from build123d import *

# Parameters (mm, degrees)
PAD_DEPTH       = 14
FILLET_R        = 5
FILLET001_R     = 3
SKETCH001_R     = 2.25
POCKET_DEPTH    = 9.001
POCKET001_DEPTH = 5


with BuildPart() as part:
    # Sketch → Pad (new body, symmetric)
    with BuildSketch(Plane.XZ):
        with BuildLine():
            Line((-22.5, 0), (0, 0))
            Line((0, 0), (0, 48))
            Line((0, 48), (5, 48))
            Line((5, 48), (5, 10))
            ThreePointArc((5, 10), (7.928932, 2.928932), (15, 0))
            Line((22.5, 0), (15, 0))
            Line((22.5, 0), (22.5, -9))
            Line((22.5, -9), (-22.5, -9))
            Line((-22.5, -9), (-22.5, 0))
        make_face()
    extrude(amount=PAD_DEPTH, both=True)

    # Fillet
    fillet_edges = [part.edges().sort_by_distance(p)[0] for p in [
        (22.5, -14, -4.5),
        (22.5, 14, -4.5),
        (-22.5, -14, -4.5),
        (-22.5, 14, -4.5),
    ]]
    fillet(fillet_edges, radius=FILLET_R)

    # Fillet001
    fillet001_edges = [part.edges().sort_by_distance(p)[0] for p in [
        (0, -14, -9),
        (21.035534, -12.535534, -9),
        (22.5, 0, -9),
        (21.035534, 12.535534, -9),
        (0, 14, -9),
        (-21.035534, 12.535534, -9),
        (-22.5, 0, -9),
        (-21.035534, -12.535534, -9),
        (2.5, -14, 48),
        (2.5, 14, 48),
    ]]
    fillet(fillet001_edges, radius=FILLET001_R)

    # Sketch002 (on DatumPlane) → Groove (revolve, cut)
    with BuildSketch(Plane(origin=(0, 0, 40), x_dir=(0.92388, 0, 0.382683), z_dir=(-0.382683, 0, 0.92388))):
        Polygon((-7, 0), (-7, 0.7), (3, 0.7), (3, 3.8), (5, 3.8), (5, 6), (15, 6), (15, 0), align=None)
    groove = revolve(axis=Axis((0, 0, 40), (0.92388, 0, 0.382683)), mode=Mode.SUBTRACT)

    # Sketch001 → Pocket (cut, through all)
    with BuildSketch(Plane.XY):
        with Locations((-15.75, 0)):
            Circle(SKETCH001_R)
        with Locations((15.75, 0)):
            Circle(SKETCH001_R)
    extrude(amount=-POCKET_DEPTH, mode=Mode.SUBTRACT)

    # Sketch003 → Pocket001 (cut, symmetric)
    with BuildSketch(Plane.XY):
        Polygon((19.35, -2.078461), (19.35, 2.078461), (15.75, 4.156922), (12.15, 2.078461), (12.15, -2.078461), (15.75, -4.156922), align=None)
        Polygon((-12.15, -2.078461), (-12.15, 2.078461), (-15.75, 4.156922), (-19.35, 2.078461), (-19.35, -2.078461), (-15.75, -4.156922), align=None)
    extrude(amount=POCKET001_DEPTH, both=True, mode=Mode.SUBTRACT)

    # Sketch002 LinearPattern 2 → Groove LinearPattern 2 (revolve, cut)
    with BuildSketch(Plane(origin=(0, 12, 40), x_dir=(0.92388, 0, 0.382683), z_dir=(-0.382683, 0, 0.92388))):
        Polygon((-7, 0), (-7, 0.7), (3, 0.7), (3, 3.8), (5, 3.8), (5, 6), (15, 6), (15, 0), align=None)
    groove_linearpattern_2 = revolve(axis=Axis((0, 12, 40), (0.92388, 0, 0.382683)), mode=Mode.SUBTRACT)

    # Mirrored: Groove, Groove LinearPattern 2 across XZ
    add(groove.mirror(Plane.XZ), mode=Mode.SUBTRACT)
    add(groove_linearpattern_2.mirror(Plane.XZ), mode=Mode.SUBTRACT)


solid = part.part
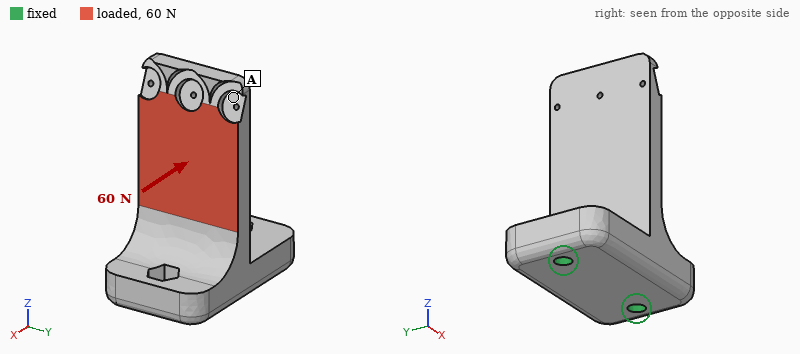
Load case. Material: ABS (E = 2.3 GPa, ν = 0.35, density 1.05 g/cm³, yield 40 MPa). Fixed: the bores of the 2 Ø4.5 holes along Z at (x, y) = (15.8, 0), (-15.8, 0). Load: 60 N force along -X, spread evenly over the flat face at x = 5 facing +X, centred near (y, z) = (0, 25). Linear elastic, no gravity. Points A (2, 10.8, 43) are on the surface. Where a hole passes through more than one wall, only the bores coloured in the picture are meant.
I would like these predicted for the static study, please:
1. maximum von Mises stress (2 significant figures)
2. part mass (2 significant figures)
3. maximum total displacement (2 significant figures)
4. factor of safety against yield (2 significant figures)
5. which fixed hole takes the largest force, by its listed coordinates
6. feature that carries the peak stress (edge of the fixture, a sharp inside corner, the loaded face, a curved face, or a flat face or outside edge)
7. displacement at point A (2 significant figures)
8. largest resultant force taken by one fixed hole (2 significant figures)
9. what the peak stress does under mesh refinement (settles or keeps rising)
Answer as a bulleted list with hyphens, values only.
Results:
- 7.7 MPa
- 18 g
- 0.88 mm
- 5.2
- (-15.8, 0)
- a curved face
- 0.75 mm
- 79 N
- settles
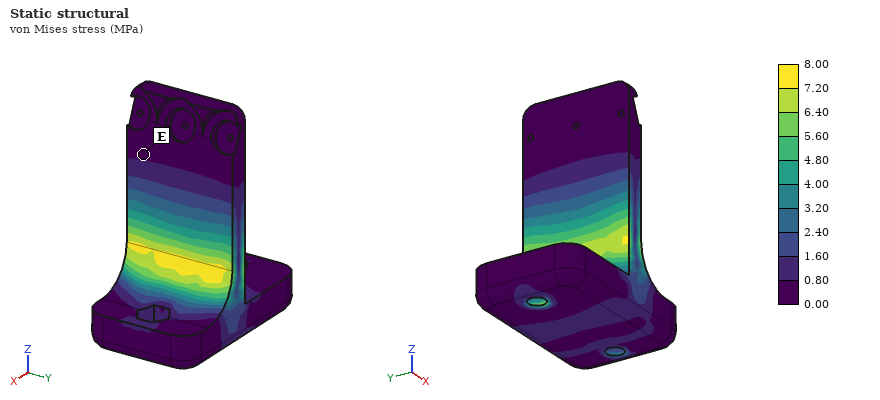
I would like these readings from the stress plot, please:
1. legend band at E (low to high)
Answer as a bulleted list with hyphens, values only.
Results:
- 0.00 to 0.80 MPa
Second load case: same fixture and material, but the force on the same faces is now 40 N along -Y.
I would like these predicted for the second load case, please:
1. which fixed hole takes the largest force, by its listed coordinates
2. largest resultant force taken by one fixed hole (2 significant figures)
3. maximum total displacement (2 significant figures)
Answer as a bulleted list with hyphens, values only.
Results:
- (15.8, 0)
- 26 N
- 0.32 mm
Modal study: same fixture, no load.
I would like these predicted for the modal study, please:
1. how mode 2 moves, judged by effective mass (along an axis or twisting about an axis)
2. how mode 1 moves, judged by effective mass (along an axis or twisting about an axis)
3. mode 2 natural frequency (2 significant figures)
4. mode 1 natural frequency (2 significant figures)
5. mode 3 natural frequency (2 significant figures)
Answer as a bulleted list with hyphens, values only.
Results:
- along Y
- along X
- 850 Hz
- 670 Hz
- 2100 Hz
